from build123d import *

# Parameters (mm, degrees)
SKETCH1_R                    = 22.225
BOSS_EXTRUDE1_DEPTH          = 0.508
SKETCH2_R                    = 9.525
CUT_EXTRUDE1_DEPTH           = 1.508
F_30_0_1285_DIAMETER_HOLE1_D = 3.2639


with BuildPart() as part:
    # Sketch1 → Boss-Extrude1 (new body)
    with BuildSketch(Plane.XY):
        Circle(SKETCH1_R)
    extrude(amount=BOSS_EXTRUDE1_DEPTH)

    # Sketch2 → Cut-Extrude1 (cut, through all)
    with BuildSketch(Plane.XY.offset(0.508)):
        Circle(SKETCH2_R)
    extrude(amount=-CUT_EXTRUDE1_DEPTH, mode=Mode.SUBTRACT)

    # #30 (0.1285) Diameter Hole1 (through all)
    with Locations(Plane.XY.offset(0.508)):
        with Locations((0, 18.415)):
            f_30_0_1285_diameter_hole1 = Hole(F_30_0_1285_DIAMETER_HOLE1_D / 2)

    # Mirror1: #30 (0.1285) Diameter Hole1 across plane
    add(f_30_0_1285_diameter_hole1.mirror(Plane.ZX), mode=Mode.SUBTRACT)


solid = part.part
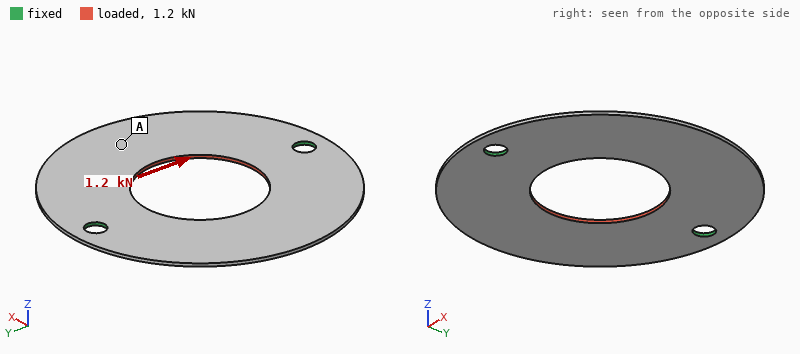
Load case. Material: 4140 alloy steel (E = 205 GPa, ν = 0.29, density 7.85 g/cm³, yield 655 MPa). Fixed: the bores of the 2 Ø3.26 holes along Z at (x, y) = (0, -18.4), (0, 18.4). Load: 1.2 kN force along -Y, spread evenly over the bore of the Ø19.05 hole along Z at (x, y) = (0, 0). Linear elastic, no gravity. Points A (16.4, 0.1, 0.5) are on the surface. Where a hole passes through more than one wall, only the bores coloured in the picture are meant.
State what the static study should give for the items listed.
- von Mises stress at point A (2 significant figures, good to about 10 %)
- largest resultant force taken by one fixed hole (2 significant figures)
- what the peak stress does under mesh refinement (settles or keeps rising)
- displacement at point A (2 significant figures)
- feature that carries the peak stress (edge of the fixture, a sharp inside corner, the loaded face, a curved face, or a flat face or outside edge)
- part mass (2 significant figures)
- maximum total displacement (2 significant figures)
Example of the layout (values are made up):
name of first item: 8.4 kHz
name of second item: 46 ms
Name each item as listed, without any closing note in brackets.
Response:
von Mises stress at point A: 20 MPa
largest resultant force taken by one fixed hole: 600 N
what the peak stress does under mesh refinement: keeps rising
displacement at point A: 6.9 µm
feature that carries the peak stress: edge of the fixture
part mass: 5.0 g
maximum total displacement: 9.3 µm
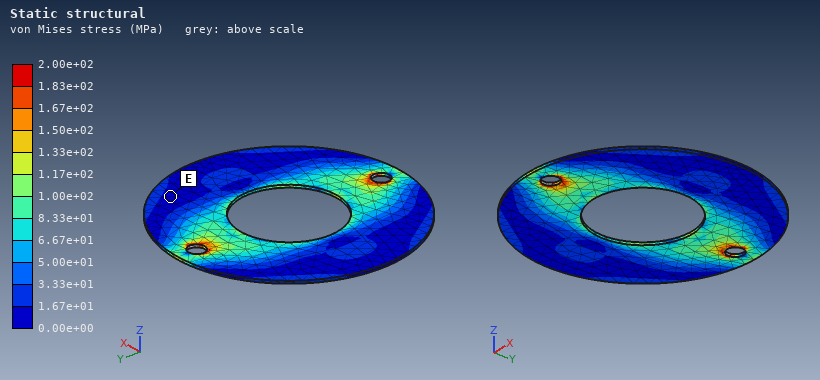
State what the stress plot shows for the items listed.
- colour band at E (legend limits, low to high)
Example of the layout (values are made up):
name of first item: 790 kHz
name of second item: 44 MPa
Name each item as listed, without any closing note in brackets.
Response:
colour band at E: 0.00e+00 to 1.67e+01 MPa
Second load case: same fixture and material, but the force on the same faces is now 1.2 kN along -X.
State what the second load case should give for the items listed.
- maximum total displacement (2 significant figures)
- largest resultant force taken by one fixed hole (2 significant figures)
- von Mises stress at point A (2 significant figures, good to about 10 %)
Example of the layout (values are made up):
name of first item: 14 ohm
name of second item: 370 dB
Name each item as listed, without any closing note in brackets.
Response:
maximum total displacement: 9.5 µm
largest resultant force taken by one fixed hole: 600 N
von Mises stress at point A: 46 MPa
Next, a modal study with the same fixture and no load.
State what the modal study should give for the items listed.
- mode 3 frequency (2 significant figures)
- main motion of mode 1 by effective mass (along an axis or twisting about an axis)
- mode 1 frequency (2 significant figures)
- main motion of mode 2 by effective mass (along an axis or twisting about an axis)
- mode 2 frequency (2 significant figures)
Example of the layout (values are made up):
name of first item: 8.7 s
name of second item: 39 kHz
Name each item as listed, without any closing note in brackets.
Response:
mode 3 frequency: 2200 Hz
main motion of mode 1 by effective mass: twisting about Y
mode 1 frequency: 780 Hz
main motion of mode 2 by effective mass: along Z
mode 2 frequency: 860 Hz
